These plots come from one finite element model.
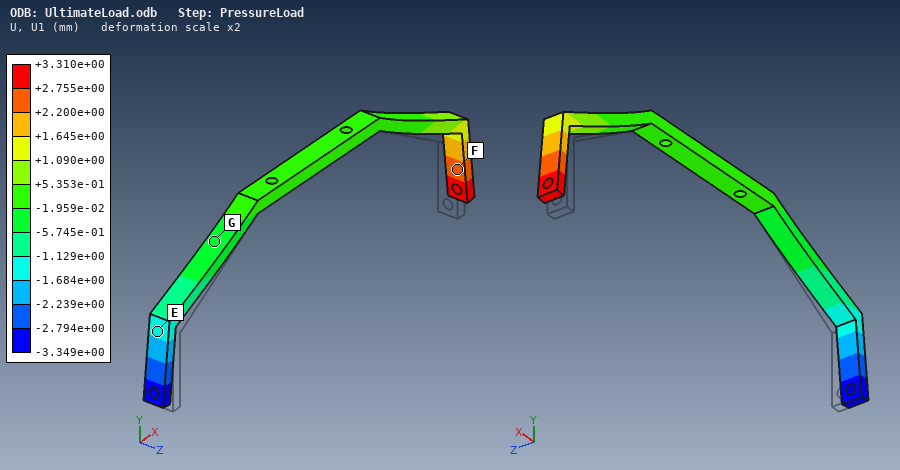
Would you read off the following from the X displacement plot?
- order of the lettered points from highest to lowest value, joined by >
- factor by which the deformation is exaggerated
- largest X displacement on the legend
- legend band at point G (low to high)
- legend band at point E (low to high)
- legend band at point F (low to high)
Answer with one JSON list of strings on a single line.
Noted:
["F > G > E", "2", "+3.310e+00 mm", "-5.745e-01 to -1.959e-02 mm", "-1.684e+00 to -1.129e+00 mm", "+2.200e+00 to +2.755e+00 mm"]
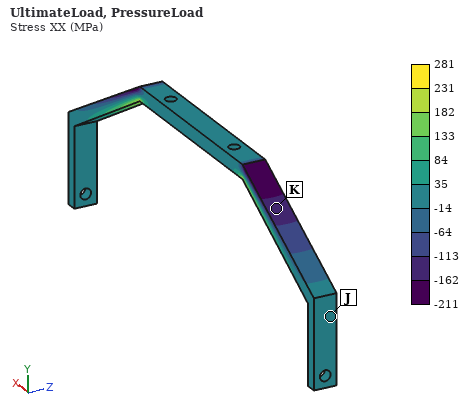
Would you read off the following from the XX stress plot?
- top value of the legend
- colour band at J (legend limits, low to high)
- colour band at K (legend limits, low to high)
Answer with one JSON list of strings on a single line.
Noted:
["281 MPa", "-14 to 35 MPa", "-162 to -113 MPa"]
